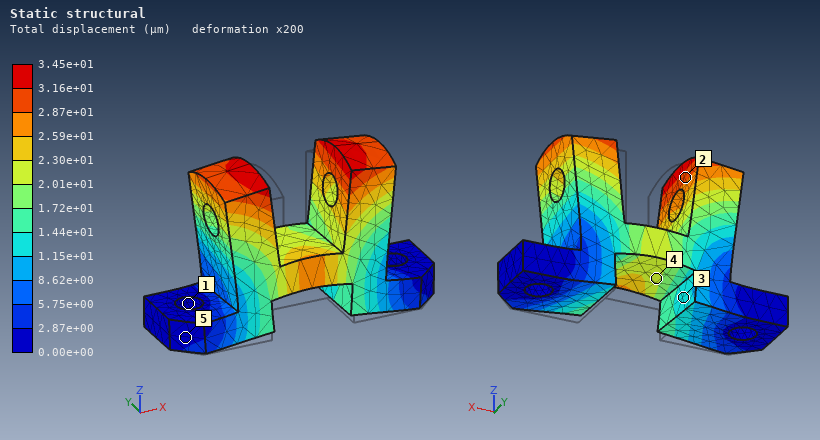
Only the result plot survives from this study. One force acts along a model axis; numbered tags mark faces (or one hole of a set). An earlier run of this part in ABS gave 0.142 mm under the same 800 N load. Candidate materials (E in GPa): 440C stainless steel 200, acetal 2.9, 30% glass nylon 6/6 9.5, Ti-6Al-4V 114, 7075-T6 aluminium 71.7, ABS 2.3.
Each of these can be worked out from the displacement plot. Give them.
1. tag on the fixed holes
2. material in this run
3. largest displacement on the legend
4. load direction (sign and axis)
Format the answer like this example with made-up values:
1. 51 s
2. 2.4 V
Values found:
1. 1
2. 30% glass nylon 6/6
3. 3.45e+01 µm
4. +Z
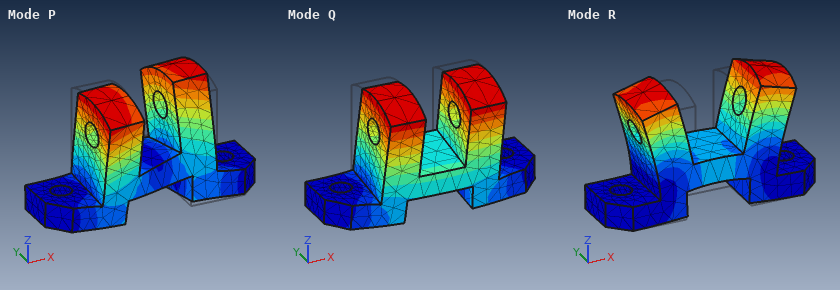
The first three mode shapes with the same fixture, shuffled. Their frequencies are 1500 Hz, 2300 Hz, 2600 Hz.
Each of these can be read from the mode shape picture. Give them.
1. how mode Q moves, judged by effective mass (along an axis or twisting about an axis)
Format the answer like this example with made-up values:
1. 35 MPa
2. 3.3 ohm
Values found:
1. along Y
